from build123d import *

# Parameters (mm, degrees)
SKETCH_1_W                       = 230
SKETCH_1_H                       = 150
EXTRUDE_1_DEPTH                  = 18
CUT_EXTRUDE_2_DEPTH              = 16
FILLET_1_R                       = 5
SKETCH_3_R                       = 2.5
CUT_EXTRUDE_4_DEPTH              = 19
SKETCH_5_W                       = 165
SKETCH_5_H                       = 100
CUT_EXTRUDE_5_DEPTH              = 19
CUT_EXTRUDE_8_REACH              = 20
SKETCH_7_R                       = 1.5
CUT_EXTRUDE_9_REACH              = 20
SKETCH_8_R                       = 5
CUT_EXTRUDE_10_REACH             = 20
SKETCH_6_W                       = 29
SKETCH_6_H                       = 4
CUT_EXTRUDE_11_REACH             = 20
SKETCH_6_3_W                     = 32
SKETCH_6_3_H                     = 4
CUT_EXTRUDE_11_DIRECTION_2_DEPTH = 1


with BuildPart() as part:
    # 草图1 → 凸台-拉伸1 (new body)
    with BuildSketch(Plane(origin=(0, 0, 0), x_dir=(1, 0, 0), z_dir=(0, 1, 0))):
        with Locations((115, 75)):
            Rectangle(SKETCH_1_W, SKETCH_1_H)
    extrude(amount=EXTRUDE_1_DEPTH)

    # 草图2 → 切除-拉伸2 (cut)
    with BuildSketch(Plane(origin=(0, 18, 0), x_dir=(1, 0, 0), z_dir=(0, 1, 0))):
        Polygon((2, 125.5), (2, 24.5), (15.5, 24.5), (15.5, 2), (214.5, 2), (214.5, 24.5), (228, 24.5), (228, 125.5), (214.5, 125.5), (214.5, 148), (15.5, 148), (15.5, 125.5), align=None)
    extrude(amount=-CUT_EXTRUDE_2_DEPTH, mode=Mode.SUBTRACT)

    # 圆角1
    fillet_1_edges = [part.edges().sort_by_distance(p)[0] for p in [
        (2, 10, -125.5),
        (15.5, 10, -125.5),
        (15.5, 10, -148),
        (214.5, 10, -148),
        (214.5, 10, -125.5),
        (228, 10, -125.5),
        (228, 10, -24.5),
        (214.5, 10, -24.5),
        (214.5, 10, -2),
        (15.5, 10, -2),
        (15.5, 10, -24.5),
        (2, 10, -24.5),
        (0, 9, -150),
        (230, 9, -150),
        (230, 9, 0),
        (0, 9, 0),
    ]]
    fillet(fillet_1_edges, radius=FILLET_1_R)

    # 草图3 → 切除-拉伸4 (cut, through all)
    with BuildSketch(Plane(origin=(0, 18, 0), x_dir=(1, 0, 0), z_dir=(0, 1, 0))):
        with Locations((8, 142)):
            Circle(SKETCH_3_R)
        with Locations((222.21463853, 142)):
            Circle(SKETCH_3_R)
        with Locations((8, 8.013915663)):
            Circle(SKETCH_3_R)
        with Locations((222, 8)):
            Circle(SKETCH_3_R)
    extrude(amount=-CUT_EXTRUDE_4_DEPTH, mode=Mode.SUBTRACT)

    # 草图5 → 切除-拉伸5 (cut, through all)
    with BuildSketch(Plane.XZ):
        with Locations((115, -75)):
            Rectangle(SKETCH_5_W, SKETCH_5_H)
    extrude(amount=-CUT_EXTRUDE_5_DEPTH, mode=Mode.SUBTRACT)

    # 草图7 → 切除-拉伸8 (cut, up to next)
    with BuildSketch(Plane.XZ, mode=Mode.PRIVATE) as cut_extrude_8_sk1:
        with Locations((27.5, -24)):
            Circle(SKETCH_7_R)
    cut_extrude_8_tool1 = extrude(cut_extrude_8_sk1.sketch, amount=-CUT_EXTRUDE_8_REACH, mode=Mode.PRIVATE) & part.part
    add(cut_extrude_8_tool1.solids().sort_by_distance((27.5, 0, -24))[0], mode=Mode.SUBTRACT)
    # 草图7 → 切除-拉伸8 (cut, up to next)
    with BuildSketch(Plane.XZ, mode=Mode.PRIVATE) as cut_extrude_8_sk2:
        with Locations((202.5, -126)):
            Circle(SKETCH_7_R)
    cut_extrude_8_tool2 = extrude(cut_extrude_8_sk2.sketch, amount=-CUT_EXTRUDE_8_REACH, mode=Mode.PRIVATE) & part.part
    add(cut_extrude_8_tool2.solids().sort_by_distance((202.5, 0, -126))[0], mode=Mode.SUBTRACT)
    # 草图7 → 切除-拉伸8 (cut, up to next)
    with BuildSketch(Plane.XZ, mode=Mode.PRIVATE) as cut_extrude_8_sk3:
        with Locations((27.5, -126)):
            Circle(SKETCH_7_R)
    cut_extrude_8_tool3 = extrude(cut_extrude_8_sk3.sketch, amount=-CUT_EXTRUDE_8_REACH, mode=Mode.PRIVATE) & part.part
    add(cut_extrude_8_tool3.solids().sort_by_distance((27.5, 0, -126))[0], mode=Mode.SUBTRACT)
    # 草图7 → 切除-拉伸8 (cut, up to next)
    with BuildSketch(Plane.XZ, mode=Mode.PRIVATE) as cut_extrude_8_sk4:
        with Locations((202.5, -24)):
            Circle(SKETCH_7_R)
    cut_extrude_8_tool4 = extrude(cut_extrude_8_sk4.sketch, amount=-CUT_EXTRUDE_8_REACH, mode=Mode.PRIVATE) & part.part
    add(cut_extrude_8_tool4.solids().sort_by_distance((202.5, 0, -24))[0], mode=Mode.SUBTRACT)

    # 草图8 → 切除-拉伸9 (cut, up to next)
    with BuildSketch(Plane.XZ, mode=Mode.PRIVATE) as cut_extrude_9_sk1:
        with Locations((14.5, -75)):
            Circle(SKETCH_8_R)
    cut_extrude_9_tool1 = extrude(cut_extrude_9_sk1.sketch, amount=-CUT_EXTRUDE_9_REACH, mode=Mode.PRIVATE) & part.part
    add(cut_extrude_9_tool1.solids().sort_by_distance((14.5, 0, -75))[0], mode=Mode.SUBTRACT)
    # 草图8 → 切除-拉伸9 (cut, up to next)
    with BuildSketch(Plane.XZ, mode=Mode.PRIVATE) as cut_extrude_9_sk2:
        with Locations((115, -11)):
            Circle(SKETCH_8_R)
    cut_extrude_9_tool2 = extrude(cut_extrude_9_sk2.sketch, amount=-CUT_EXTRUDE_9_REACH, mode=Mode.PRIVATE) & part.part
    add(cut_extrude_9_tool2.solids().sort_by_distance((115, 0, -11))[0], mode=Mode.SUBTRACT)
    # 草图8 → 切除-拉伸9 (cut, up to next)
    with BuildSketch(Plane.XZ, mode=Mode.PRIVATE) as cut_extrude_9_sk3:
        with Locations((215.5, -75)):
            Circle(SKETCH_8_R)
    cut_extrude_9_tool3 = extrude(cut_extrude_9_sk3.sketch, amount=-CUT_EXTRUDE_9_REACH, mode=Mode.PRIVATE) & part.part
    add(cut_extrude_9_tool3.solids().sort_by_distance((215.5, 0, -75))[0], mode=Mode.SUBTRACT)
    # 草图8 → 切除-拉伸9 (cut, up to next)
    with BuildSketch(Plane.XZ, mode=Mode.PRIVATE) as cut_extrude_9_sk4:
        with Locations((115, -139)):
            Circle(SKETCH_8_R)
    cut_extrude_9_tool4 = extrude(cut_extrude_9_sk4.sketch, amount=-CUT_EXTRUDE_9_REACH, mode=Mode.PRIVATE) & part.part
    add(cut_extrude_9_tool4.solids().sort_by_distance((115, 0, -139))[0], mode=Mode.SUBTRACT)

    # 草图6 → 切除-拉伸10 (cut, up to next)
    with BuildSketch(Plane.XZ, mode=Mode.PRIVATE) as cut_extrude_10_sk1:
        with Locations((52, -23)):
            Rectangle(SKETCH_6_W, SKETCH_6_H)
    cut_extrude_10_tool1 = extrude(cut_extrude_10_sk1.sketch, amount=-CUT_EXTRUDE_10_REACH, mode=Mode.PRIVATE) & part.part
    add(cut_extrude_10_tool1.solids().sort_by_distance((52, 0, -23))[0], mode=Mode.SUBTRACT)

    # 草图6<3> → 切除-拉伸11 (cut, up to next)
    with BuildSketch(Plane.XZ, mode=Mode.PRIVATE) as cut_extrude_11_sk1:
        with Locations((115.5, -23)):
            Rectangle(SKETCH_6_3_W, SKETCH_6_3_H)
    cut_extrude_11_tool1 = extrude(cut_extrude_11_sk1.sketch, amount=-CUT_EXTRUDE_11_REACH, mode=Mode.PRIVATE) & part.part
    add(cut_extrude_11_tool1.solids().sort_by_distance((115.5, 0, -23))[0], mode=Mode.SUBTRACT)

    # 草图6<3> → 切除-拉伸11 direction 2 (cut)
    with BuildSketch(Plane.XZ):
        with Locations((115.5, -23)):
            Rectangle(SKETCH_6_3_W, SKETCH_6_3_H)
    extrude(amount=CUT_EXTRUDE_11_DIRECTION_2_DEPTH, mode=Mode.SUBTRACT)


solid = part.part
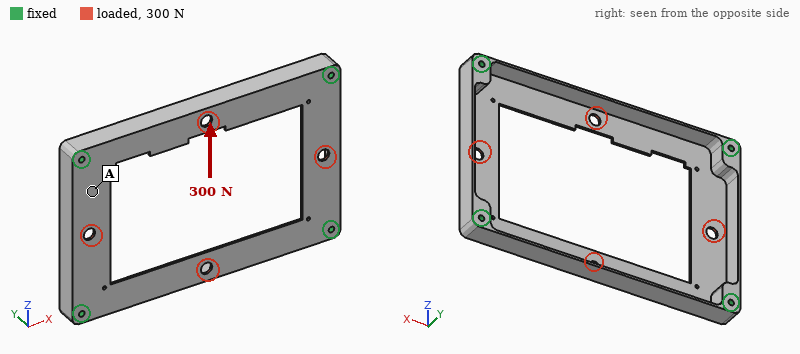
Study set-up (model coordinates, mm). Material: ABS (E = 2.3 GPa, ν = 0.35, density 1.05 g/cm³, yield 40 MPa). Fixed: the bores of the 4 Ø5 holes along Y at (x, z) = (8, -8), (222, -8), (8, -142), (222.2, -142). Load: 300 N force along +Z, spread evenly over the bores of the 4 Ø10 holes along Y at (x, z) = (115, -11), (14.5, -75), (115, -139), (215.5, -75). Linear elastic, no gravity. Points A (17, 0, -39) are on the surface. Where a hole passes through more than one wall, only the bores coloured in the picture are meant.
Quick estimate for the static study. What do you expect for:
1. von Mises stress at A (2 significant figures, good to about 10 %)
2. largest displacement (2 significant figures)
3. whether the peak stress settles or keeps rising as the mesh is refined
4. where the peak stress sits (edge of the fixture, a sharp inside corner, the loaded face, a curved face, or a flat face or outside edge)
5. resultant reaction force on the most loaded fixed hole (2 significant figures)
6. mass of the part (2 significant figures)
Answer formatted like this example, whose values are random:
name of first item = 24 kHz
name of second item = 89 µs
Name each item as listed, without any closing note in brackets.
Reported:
von Mises stress at A = 1.0 MPa
largest displacement = 0.72 mm
whether the peak stress settles or keeps rising as the mesh is refined = keeps rising
where the peak stress sits = a sharp inside corner
resultant reaction force on the most loaded fixed hole = 81 N
mass of the part = 81 g
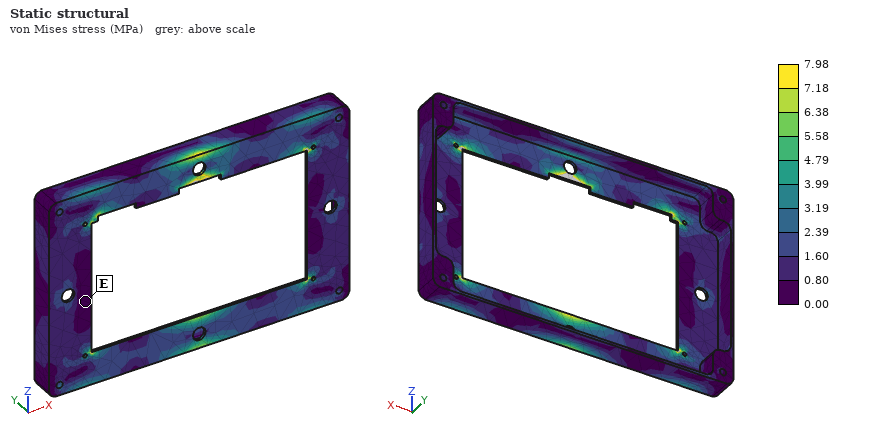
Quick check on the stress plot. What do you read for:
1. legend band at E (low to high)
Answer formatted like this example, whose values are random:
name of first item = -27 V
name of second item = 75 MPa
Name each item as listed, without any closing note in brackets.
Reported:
legend band at E = 0.00 to 0.80 MPa
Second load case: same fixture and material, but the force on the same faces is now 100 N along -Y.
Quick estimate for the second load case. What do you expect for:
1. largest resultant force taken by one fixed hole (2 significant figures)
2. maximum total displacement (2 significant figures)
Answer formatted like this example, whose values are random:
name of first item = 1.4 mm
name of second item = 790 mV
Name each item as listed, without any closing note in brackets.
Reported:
largest resultant force taken by one fixed hole = 26 N
maximum total displacement = 2.8 mm
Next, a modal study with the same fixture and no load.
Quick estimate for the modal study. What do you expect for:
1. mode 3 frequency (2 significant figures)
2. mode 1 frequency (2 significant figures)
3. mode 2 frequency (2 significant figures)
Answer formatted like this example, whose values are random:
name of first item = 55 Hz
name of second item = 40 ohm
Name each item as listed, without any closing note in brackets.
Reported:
mode 3 frequency = 400 Hz
mode 1 frequency = 250 Hz
mode 2 frequency = 260 Hz
